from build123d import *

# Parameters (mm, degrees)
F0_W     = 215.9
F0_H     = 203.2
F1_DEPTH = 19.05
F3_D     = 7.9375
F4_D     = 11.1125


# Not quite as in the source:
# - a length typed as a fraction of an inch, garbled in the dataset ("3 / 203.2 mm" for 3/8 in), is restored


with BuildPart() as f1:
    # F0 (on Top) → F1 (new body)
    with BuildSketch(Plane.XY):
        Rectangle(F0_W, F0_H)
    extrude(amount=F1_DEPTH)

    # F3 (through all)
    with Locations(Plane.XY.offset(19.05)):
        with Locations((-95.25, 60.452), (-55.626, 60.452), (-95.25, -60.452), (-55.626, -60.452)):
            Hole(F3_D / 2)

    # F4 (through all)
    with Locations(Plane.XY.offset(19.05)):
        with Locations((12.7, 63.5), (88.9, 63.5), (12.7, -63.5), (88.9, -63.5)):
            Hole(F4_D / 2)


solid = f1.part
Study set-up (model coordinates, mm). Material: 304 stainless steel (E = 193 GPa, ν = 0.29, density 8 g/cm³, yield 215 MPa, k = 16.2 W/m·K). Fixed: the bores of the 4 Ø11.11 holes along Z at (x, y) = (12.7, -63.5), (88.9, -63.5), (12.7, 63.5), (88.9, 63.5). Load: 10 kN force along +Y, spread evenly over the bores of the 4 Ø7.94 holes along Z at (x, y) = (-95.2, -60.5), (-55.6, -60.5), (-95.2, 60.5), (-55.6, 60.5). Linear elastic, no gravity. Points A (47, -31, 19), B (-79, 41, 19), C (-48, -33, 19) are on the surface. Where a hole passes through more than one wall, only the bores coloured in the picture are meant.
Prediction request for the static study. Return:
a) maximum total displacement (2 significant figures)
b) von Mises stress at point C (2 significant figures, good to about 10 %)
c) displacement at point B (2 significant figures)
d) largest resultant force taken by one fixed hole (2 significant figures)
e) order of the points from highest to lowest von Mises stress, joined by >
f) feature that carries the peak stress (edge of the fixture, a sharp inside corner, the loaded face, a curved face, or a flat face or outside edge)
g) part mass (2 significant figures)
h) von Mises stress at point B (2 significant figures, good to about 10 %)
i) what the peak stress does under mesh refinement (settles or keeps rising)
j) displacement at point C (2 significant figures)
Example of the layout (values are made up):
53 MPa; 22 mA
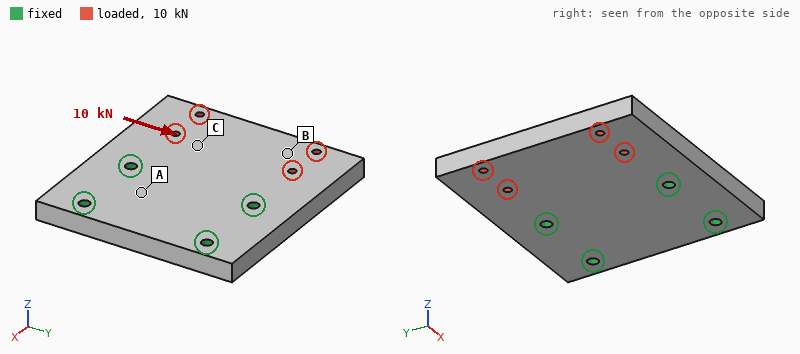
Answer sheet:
7.5 µm; 5.9 MPa; 5.5 µm; 7.2 kN; C > B > A; edge of the fixture; 6.6 kg; 3.3 MPa; keeps rising; 3.8 µm
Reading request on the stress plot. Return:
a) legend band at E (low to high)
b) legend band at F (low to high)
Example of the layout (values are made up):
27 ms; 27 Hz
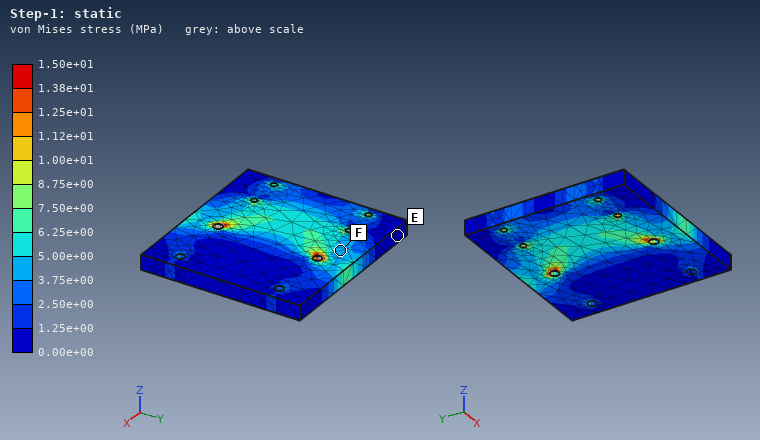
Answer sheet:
0.00e+00 to 1.25e+00 MPa; 3.75e+00 to 5.00e+00 MPa
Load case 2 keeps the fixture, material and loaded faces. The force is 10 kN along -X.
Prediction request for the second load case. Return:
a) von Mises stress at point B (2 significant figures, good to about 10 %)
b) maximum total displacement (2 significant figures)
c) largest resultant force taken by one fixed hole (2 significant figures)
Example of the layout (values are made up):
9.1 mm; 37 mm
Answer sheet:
3.0 MPa; 2.3 µm; 3.9 kN
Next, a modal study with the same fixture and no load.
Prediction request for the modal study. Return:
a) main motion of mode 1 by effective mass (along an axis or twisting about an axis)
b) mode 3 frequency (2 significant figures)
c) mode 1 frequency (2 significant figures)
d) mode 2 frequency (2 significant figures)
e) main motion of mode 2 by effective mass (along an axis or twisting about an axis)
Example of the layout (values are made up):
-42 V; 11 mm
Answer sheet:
along Z; 3100 Hz; 920 Hz; 1600 Hz; twisting about X
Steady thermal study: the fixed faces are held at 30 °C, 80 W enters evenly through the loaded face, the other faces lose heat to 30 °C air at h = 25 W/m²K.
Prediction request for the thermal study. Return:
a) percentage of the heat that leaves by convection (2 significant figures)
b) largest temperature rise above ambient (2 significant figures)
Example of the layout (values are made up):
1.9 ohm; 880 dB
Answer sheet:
68 %; 77 K
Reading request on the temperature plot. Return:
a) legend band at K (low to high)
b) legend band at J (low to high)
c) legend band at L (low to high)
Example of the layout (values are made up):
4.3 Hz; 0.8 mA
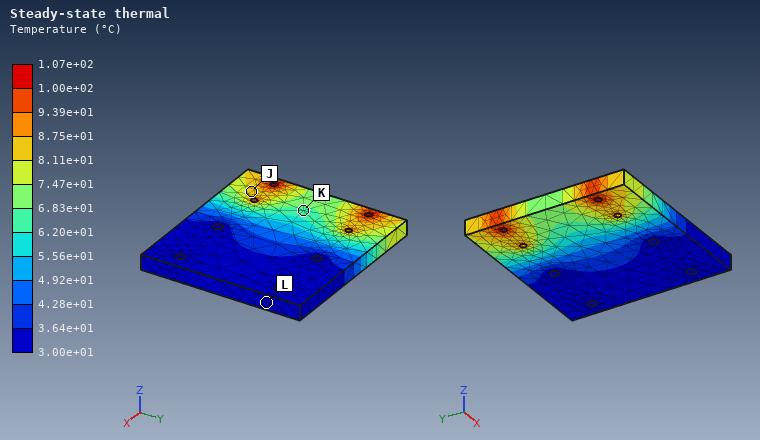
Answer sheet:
6.20e+01 to 6.83e+01 °C; 8.11e+01 to 8.75e+01 °C; 3.00e+01 to 3.64e+01 °C
